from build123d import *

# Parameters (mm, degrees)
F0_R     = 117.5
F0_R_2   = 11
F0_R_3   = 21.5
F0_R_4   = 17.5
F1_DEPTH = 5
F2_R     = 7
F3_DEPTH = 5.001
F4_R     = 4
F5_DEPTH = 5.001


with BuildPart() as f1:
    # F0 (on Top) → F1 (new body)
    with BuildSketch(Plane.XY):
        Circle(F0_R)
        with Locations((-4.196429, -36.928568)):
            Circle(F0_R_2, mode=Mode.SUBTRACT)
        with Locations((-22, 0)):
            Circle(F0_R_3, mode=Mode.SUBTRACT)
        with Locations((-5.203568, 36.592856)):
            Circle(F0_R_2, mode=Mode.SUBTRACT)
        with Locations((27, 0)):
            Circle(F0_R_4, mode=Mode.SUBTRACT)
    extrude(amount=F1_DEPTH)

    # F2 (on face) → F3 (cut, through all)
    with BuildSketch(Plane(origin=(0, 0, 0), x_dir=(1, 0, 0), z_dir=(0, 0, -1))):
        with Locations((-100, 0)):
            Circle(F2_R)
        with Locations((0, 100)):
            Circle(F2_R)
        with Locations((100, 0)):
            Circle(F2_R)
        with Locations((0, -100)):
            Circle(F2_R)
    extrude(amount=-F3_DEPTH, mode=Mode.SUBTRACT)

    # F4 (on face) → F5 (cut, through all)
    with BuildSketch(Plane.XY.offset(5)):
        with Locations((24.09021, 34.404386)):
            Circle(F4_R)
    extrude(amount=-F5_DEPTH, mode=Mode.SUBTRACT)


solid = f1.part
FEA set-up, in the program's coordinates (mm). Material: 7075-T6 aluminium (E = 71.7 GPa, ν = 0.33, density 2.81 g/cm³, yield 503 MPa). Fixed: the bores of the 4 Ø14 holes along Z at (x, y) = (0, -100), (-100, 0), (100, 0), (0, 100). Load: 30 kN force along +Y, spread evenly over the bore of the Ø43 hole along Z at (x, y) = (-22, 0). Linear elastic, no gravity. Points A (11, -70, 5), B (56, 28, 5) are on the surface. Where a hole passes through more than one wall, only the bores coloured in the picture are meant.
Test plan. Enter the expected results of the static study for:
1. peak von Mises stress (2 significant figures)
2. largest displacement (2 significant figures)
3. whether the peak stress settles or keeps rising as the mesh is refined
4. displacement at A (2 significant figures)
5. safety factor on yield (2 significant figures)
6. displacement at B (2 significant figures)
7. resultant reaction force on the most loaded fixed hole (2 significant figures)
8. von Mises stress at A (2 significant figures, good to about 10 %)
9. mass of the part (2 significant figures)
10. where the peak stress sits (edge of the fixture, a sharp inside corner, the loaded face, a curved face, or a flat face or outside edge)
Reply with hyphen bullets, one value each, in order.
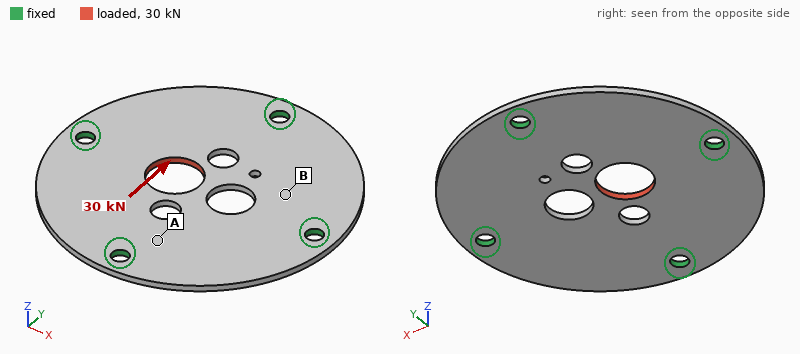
- 160 MPa
- 79 µm
- settles
- 15 µm
- 3.1
- 13 µm
- 9.0 kN
- 32 MPa
- 560 g
- a curved face
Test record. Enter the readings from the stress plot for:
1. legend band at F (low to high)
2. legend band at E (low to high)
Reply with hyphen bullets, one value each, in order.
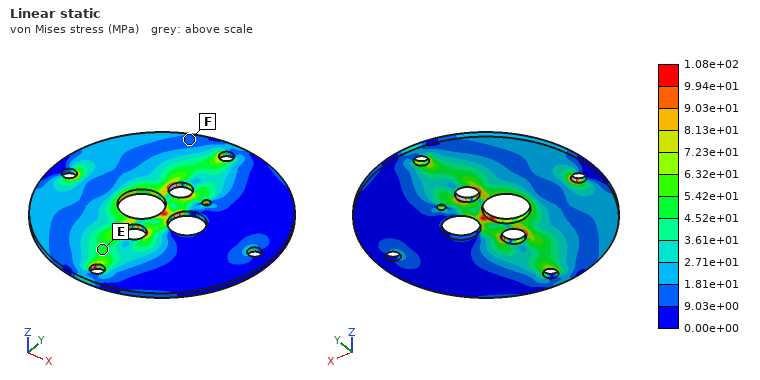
- 9.03e+00 to 1.81e+01 MPa
- 4.52e+01 to 5.42e+01 MPa
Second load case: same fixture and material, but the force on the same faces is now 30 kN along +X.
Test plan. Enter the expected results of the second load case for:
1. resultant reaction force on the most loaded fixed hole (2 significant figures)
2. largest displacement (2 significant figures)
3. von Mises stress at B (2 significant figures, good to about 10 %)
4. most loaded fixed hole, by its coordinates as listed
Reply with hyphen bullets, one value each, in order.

- 13 kN
- 93 µm
- 31 MPa
- (-100, 0)
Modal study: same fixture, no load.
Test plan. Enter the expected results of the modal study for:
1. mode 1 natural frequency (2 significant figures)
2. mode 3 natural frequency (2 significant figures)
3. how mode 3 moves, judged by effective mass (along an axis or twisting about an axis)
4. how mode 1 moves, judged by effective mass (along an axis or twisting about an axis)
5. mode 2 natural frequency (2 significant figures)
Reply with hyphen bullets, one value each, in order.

- 1100 Hz
- 1200 Hz
- twisting about X
- along Z
- 1100 Hz
